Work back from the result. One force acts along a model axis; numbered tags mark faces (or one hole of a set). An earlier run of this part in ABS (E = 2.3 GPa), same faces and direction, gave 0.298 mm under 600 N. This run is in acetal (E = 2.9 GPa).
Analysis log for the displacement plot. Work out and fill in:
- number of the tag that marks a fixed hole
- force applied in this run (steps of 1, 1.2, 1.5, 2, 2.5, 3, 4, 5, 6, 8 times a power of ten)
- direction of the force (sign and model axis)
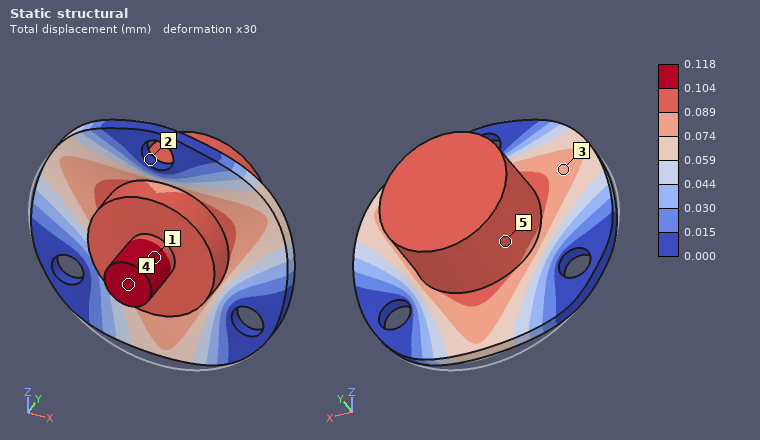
2
300 N
+Y
